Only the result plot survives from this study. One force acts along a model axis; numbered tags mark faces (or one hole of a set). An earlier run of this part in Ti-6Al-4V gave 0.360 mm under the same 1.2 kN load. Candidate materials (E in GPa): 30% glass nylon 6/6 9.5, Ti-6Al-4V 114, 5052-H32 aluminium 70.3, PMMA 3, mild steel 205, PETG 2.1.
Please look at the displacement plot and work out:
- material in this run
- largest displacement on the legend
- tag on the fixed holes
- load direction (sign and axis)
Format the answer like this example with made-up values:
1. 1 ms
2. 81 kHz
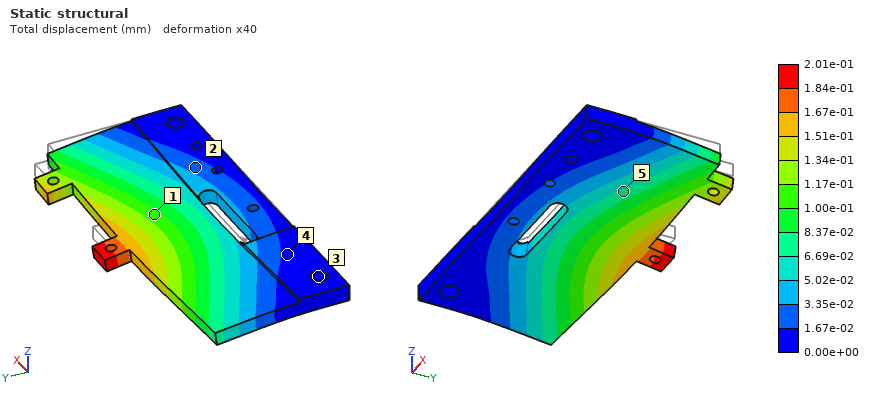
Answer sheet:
1. mild steel
2. 2.01e-01 mm
3. 3
4. -Z
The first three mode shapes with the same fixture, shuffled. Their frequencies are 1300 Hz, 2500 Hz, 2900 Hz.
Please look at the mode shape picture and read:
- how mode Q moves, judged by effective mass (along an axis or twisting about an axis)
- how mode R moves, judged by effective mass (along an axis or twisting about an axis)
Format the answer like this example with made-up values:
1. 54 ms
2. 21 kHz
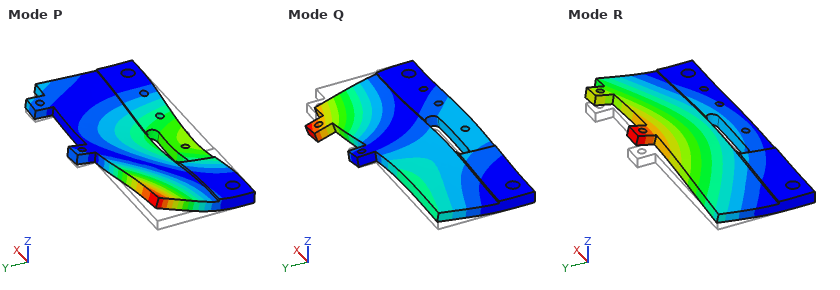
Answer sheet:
1. twisting about Y
2. along Z
